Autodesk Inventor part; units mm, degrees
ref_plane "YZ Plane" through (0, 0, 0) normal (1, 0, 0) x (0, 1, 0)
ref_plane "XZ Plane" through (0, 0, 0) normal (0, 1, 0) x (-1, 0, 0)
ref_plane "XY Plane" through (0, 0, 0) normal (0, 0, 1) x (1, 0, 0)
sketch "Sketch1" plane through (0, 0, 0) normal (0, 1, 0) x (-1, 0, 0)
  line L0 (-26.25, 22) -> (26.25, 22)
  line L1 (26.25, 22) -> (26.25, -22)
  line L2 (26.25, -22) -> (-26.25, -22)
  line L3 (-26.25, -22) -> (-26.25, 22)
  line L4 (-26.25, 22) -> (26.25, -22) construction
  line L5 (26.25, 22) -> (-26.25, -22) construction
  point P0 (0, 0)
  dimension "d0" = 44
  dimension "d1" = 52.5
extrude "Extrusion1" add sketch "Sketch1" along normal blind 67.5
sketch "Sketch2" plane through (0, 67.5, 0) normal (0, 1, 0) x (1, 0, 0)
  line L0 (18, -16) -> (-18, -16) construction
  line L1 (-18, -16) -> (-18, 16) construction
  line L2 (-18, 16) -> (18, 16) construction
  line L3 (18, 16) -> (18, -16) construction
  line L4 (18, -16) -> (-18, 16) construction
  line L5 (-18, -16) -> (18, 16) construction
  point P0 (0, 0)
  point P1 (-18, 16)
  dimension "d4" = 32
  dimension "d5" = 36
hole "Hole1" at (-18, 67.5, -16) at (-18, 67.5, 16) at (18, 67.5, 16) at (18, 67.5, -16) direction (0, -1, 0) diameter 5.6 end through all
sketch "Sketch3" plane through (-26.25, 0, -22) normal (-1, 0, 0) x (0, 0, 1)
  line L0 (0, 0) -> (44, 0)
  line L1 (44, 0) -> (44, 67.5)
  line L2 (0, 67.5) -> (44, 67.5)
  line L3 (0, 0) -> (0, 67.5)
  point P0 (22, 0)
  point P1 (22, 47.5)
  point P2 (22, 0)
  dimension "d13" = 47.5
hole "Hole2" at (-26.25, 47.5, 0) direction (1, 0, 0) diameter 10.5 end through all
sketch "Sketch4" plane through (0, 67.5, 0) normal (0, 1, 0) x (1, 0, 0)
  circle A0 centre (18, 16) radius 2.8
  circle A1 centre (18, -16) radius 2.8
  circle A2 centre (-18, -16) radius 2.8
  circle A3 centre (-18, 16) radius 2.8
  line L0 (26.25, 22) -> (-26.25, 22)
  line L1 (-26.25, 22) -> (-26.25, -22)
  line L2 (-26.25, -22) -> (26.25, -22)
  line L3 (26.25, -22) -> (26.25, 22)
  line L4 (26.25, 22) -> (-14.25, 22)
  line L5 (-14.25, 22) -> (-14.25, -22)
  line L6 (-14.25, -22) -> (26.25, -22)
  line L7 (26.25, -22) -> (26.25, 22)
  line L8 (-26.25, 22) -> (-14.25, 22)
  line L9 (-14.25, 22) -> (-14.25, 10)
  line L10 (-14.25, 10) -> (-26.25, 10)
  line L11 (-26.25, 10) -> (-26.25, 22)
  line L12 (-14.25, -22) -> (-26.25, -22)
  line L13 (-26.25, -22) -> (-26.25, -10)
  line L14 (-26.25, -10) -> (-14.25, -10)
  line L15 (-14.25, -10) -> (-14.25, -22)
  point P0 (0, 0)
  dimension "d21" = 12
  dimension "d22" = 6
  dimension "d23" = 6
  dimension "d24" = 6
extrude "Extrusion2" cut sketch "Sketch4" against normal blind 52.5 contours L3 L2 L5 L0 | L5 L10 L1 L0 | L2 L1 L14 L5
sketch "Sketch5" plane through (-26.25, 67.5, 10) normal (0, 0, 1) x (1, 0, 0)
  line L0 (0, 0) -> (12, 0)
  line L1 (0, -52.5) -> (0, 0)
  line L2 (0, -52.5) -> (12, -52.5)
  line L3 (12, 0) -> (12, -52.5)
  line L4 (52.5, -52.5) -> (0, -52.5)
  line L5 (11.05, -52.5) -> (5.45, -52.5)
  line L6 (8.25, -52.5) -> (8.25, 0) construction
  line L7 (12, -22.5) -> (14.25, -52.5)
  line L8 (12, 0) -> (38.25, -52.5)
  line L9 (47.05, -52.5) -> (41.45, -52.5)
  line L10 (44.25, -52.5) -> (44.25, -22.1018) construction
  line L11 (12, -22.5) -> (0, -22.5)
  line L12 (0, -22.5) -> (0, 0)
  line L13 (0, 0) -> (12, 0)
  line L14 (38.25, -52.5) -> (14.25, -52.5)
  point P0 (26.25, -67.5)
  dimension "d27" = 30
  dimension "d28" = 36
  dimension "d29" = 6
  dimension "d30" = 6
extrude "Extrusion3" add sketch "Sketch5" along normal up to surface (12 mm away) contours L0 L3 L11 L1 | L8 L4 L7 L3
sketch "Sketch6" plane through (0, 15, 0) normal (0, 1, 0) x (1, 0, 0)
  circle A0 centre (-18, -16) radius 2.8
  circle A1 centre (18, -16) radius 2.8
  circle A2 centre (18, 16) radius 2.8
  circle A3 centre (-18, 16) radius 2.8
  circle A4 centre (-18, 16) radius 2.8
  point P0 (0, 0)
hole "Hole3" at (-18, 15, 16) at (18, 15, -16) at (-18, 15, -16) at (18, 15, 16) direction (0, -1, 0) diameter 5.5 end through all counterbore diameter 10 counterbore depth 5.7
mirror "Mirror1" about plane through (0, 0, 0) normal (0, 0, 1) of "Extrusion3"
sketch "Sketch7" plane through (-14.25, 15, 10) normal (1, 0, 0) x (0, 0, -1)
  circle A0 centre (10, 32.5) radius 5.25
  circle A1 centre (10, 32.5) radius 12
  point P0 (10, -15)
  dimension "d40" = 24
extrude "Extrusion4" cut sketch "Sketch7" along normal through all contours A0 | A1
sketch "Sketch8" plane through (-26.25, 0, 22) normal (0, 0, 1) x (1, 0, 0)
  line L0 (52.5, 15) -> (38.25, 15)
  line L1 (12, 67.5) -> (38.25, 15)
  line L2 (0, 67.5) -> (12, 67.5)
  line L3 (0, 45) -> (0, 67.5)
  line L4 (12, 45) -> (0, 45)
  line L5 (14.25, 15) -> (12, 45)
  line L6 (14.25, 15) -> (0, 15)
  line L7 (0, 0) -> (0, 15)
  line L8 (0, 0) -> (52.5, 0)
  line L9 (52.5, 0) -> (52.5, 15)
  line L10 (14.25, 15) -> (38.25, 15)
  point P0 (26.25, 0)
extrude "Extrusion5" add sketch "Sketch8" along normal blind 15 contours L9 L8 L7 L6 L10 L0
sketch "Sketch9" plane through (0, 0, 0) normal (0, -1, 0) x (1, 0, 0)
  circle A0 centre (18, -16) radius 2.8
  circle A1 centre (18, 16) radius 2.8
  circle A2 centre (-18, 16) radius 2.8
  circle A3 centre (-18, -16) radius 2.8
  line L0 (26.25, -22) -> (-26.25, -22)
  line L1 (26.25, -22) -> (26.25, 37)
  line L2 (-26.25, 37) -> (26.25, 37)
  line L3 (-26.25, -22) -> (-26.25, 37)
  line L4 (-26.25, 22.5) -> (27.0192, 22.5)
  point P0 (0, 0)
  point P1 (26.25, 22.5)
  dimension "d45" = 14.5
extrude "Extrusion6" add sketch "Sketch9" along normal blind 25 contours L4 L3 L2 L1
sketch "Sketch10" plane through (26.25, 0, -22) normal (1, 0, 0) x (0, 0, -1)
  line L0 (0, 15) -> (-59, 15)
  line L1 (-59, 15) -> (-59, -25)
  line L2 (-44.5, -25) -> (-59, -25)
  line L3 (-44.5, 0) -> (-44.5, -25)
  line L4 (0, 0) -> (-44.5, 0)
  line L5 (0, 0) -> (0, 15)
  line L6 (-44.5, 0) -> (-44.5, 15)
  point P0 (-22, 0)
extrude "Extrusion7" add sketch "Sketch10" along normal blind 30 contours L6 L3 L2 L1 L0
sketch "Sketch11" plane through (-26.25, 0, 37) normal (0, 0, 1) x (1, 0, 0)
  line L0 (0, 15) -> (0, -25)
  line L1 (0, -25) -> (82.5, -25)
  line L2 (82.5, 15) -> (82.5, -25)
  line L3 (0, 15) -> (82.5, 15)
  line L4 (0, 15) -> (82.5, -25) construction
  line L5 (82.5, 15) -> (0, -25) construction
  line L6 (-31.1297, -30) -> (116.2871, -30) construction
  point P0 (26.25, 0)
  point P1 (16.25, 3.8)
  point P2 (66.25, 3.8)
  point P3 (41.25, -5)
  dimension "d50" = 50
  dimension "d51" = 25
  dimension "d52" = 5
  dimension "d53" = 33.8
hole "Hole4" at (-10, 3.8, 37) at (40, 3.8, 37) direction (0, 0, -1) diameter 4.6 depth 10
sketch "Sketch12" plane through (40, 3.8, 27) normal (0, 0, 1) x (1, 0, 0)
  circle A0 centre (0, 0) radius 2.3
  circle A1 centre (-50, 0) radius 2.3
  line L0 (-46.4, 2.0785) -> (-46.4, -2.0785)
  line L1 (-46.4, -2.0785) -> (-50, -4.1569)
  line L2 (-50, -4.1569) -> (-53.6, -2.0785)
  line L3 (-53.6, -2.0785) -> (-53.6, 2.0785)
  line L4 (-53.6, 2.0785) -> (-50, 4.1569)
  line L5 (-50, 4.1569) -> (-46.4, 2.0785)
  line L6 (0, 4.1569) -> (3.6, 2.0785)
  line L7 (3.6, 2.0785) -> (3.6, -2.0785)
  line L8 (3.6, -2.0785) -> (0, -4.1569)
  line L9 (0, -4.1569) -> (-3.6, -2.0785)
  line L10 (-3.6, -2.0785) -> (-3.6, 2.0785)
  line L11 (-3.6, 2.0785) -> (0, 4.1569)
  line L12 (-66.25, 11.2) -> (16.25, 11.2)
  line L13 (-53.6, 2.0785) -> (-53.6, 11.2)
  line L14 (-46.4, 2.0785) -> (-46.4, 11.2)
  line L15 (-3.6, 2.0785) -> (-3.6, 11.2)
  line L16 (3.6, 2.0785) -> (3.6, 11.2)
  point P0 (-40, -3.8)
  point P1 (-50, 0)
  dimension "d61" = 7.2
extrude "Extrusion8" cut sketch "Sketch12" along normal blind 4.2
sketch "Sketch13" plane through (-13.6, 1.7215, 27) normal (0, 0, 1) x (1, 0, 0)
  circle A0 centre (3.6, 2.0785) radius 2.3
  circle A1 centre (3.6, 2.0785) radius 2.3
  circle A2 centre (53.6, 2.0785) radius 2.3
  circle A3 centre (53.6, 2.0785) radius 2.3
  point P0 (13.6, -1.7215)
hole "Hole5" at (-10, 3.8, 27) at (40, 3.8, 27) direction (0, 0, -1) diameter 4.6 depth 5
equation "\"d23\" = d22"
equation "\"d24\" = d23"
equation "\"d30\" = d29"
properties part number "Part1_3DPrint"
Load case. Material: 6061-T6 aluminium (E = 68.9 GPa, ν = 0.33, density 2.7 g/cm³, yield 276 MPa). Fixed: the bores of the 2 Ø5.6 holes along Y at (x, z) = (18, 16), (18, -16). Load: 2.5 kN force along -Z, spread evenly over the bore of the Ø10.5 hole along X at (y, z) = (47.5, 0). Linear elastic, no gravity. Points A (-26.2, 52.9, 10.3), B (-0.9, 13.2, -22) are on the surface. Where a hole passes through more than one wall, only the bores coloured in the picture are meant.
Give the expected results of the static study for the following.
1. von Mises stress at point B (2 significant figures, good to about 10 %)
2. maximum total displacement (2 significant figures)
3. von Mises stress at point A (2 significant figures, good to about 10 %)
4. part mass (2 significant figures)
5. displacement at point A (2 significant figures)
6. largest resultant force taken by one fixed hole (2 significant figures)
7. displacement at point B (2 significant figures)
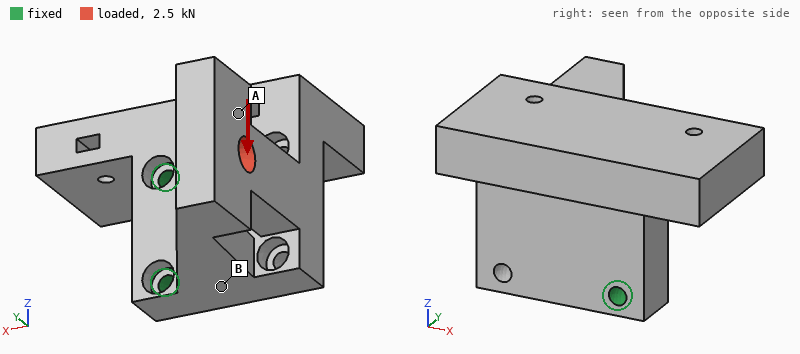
24 MPa
0.11 mm
8.3 MPa
300 g
0.082 mm
4.2 kN
0.022 mm
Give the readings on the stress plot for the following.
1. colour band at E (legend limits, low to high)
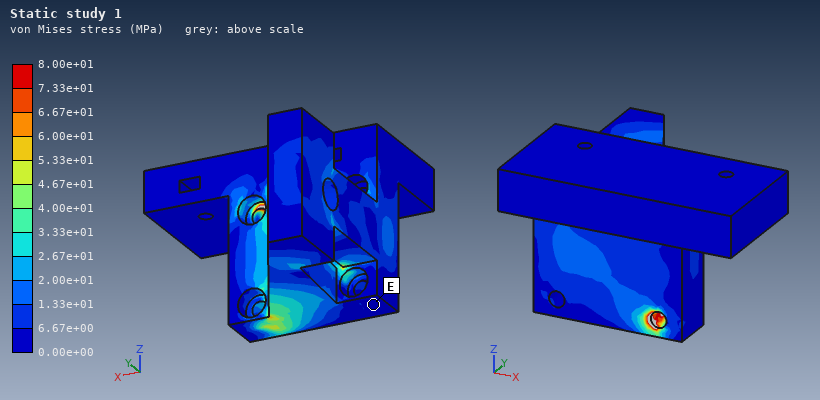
0.00e+00 to 6.67e+00 MPa
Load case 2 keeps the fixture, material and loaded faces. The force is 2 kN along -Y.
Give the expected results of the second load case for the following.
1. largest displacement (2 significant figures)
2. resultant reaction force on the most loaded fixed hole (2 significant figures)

0.17 mm
1.0 kN
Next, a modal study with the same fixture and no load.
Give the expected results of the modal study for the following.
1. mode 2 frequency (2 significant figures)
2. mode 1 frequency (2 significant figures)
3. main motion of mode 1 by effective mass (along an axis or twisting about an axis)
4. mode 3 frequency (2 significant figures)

3000 Hz
1600 Hz
along Y
4300 Hz
